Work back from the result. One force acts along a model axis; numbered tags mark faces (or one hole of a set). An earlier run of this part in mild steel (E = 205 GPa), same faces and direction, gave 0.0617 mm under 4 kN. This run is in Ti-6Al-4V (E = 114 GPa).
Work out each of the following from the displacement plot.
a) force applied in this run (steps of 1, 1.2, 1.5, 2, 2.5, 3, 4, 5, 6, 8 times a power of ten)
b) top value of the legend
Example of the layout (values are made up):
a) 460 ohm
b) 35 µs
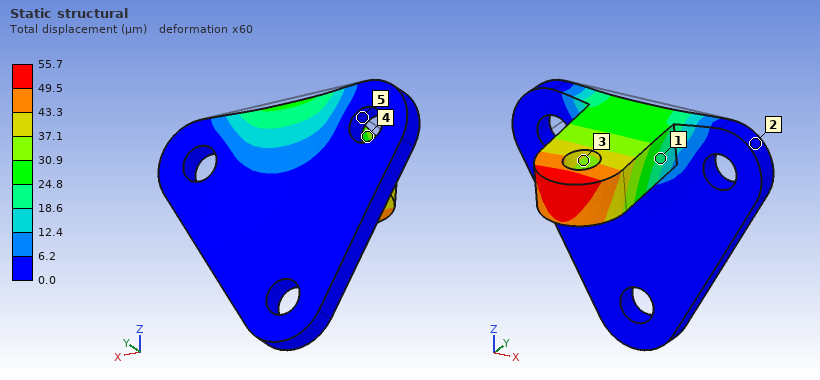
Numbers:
a) 2 kN
b) 55.7 µm
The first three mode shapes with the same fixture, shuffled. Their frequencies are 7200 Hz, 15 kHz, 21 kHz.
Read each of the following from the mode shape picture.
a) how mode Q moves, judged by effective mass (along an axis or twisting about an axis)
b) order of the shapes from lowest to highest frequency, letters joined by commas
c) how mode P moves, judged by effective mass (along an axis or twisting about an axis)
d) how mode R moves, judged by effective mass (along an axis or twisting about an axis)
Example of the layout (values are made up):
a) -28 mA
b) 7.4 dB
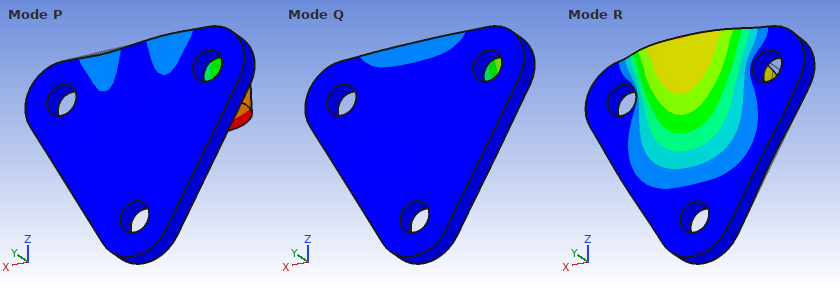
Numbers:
a) along Z
b) Q, P, R
c) along X
d) along Y
